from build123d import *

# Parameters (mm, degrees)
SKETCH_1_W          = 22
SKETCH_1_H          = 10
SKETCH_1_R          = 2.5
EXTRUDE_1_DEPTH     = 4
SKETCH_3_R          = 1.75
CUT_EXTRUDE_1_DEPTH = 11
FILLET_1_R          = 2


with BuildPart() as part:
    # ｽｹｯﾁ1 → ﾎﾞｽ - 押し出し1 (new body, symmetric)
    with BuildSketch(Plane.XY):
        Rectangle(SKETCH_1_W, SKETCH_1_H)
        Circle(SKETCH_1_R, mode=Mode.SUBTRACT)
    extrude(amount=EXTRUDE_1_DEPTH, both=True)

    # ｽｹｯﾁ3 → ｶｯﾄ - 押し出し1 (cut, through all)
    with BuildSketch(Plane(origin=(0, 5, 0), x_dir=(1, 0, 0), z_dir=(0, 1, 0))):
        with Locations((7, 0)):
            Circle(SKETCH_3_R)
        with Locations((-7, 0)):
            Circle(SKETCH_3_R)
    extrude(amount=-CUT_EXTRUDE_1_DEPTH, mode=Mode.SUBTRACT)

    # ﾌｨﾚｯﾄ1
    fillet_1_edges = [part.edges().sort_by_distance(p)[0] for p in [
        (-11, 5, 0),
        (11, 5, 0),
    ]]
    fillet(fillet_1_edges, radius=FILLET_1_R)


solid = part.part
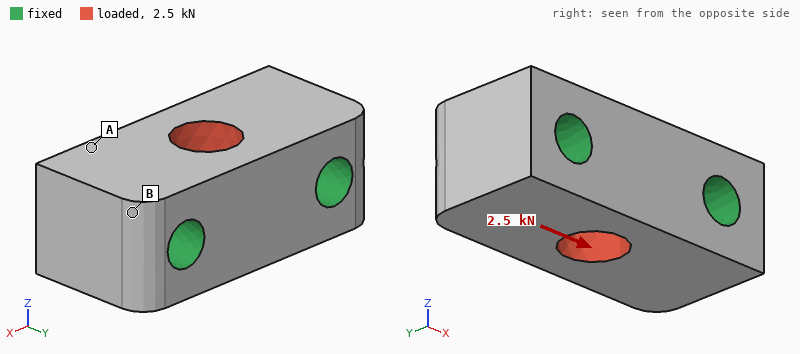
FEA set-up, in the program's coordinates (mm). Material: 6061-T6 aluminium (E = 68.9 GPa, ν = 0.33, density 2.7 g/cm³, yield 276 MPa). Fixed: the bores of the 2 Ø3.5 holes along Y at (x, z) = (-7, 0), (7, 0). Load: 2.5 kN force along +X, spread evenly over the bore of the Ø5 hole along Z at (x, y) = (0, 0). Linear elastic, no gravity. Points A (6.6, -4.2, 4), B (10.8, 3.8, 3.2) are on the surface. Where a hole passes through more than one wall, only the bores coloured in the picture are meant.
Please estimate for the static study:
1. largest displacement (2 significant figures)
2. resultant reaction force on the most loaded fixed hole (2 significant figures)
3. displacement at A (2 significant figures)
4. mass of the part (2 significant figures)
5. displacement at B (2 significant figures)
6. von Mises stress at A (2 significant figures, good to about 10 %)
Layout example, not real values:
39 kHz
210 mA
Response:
1.6 µm
1.3 kN
0.48 µm
3.8 g
0.27 µm
6.4 MPa
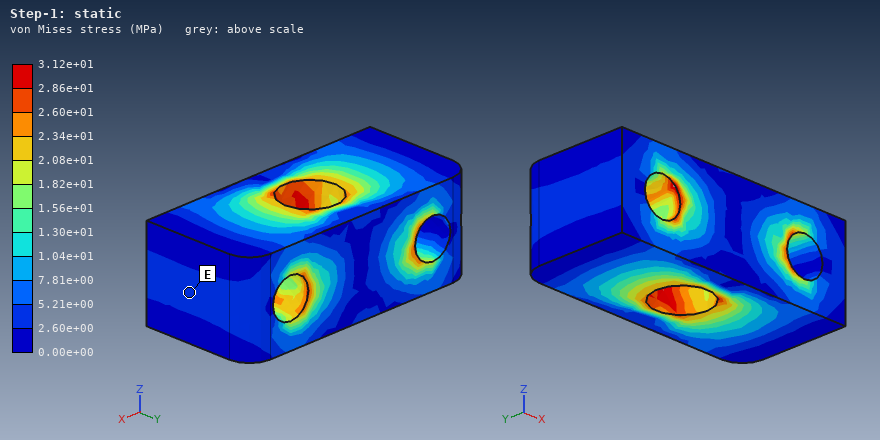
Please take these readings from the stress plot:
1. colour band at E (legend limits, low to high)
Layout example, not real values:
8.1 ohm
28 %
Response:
2.60e+00 to 5.21e+00 MPa
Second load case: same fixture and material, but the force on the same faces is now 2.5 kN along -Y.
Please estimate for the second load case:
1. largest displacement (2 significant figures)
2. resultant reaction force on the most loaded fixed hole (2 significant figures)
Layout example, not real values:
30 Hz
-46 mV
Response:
4.6 µm
1.3 kN
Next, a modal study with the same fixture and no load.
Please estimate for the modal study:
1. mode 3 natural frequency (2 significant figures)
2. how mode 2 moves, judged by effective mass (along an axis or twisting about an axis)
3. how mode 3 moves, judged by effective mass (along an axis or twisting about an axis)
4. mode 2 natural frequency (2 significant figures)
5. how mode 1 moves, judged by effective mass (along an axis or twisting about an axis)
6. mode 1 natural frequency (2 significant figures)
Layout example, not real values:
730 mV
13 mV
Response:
130 kHz
twisting about X
along Y
120 kHz
along Z
110 kHz
